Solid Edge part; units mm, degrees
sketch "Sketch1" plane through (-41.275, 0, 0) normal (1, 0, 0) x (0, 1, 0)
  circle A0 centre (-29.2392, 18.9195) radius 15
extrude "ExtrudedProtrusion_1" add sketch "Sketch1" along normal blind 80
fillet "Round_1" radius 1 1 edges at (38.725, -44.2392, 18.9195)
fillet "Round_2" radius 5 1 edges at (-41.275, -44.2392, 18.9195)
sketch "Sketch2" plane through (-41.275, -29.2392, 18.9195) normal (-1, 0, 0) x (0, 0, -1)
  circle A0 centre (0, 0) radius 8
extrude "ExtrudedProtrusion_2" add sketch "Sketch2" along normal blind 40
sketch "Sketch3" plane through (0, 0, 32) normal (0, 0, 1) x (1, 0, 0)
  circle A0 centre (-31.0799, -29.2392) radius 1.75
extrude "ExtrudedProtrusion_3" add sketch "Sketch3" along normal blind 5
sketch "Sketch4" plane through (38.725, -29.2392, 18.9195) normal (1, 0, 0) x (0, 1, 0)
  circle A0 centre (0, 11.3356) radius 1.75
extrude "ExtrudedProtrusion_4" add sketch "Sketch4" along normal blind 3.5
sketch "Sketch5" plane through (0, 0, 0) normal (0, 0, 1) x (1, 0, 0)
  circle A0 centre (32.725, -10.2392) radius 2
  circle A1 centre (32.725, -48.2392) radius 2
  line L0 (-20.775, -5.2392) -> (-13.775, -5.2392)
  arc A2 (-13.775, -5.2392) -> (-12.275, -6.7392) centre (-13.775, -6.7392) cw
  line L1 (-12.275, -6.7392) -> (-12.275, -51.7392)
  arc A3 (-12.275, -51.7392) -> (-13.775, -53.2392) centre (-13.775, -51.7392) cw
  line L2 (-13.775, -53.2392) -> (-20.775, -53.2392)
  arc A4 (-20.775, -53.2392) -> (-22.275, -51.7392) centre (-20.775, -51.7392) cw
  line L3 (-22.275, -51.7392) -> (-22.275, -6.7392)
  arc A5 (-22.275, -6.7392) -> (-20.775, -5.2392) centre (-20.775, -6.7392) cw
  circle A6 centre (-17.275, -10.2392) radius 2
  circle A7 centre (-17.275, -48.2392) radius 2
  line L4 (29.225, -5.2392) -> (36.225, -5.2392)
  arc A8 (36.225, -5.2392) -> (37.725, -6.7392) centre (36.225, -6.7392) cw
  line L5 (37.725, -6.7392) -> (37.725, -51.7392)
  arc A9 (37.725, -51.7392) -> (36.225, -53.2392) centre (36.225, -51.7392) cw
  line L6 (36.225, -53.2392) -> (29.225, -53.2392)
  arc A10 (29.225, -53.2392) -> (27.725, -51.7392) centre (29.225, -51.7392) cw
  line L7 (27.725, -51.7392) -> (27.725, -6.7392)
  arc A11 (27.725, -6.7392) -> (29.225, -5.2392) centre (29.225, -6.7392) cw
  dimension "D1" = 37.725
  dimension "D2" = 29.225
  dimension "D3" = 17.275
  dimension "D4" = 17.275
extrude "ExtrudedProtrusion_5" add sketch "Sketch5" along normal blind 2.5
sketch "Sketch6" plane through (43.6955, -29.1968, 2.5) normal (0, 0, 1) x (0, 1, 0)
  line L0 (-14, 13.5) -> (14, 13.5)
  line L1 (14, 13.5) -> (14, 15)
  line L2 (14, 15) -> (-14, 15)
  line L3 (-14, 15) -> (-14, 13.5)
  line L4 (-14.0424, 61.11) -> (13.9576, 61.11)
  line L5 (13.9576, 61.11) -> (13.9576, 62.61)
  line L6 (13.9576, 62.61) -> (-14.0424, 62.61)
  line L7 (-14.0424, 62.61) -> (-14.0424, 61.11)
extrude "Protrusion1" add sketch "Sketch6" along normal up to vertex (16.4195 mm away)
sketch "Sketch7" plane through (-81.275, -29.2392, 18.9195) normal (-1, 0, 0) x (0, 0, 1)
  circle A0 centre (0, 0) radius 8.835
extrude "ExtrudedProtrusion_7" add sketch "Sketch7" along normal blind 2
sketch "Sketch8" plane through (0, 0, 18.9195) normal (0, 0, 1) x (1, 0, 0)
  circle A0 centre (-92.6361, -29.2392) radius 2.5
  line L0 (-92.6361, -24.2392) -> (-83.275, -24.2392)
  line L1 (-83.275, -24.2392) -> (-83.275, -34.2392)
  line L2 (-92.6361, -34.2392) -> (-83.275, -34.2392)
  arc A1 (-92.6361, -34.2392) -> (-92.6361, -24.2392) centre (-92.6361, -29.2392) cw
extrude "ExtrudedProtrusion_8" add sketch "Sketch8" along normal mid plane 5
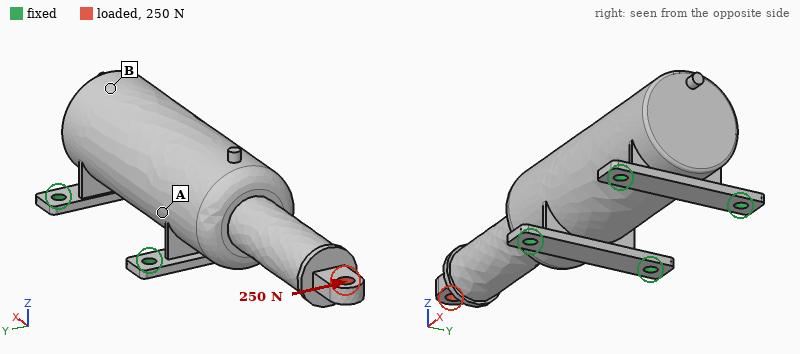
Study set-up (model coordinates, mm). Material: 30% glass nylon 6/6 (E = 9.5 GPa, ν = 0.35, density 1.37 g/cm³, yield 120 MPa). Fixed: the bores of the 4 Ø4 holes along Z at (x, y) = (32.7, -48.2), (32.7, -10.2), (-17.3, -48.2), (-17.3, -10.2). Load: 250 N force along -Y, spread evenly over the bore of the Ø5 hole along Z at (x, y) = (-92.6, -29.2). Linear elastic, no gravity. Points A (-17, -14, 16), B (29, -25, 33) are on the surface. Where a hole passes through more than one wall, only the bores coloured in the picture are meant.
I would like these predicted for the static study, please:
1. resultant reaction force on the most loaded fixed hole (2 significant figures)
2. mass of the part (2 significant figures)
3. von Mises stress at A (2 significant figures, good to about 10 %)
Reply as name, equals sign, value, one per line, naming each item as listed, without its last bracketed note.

resultant reaction force on the most loaded fixed hole = 340 N
mass of the part = 93 g
von Mises stress at A = 7.2 MPa
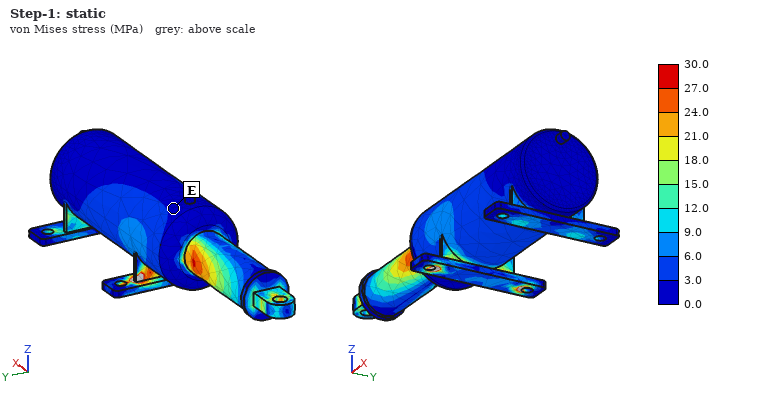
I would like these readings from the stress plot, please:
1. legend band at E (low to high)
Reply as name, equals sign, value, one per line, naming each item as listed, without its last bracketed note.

legend band at E = 0.0 to 3.0 MPa
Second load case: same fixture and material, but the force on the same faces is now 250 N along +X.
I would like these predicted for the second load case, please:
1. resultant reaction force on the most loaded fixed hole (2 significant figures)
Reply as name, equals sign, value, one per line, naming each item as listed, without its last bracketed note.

resultant reaction force on the most loaded fixed hole = 85 N
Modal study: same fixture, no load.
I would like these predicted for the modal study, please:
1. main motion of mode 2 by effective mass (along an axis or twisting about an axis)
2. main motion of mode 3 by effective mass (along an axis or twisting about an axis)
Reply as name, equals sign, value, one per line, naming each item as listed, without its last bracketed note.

main motion of mode 2 by effective mass = along Y
main motion of mode 3 by effective mass = along X
